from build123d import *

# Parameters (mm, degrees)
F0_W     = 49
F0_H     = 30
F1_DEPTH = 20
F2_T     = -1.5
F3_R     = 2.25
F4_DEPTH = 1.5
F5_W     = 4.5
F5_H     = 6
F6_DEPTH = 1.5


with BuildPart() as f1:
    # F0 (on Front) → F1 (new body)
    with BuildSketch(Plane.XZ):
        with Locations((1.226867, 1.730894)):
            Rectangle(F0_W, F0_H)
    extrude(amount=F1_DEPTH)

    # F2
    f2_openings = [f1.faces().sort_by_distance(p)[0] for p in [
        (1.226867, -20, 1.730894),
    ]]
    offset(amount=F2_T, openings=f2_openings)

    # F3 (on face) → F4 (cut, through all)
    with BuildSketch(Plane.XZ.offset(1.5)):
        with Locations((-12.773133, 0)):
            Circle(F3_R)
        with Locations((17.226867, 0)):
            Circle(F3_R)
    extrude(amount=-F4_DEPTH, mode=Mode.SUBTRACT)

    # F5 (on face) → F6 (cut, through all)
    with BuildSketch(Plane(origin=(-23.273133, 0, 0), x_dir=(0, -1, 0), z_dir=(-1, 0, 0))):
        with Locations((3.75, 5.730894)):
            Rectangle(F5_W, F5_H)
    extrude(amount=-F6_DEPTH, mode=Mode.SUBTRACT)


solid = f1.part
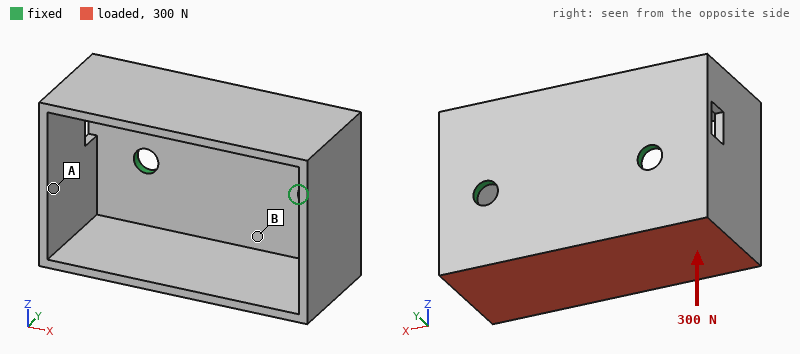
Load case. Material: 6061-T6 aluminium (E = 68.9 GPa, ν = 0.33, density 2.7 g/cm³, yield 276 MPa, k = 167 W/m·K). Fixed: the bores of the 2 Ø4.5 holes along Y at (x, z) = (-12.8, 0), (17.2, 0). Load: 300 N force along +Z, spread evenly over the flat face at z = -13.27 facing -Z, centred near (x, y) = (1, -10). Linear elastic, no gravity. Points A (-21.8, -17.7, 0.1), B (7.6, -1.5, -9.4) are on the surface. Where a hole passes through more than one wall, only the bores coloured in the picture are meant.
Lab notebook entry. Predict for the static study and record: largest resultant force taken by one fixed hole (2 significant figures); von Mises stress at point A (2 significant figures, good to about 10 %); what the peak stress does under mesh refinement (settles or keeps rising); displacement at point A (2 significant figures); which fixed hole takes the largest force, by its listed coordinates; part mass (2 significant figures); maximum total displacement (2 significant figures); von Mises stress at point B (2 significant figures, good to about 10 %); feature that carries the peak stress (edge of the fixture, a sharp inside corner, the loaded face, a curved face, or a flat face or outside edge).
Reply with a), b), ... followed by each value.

a) 160 N
b) 15 MPa
c) keeps rising
d) 0.11 mm
e) (-12.8, 0)
f) 17 g
g) 0.31 mm
h) 47 MPa
i) edge of the fixture
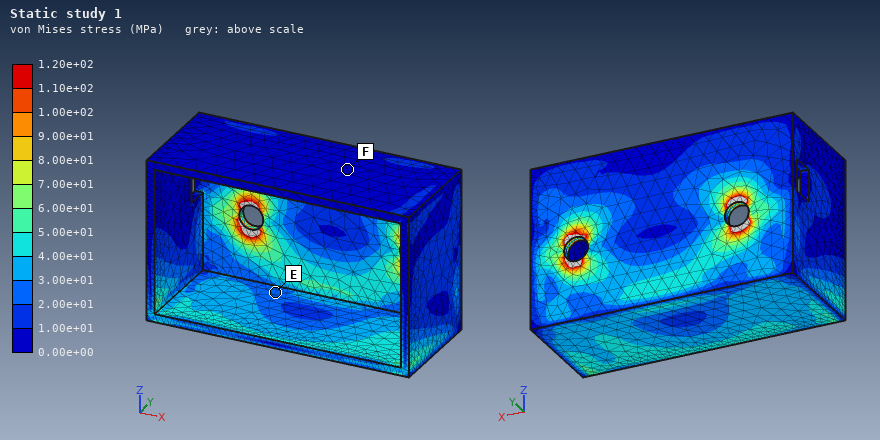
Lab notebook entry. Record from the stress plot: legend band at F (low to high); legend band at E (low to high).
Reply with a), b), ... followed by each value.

a) 0.00e+00 to 1.00e+01 MPa
b) 2.00e+01 to 3.00e+01 MPa
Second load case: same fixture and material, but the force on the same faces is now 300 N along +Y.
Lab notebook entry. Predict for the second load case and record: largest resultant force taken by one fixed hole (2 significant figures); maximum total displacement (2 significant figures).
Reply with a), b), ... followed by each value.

a) 160 N
b) 0.23 mm
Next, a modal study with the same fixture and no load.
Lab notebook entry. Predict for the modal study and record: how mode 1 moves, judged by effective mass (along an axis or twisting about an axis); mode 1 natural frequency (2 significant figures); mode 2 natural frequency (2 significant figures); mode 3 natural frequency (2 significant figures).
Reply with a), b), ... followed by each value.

a) along Z
b) 1800 Hz
c) 2500 Hz
d) 4000 Hz
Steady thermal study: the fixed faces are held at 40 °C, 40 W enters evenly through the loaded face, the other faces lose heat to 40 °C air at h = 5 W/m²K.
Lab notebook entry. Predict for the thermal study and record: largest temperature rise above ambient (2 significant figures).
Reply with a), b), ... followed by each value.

a) 59 K
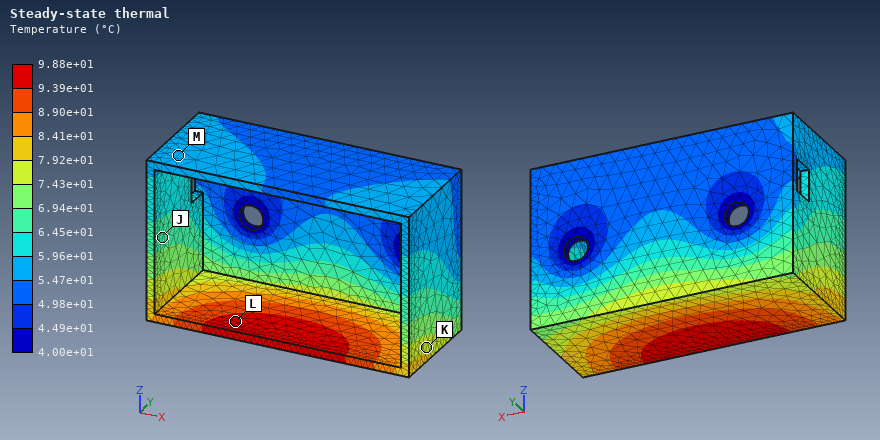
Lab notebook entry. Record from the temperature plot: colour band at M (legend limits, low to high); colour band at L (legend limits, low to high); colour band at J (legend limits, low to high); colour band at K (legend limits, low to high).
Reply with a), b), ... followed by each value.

a) 5.47e+01 to 5.96e+01 °C
b) 9.39e+01 to 9.88e+01 °C
c) 6.45e+01 to 6.94e+01 °C
d) 7.43e+01 to 7.92e+01 °C
